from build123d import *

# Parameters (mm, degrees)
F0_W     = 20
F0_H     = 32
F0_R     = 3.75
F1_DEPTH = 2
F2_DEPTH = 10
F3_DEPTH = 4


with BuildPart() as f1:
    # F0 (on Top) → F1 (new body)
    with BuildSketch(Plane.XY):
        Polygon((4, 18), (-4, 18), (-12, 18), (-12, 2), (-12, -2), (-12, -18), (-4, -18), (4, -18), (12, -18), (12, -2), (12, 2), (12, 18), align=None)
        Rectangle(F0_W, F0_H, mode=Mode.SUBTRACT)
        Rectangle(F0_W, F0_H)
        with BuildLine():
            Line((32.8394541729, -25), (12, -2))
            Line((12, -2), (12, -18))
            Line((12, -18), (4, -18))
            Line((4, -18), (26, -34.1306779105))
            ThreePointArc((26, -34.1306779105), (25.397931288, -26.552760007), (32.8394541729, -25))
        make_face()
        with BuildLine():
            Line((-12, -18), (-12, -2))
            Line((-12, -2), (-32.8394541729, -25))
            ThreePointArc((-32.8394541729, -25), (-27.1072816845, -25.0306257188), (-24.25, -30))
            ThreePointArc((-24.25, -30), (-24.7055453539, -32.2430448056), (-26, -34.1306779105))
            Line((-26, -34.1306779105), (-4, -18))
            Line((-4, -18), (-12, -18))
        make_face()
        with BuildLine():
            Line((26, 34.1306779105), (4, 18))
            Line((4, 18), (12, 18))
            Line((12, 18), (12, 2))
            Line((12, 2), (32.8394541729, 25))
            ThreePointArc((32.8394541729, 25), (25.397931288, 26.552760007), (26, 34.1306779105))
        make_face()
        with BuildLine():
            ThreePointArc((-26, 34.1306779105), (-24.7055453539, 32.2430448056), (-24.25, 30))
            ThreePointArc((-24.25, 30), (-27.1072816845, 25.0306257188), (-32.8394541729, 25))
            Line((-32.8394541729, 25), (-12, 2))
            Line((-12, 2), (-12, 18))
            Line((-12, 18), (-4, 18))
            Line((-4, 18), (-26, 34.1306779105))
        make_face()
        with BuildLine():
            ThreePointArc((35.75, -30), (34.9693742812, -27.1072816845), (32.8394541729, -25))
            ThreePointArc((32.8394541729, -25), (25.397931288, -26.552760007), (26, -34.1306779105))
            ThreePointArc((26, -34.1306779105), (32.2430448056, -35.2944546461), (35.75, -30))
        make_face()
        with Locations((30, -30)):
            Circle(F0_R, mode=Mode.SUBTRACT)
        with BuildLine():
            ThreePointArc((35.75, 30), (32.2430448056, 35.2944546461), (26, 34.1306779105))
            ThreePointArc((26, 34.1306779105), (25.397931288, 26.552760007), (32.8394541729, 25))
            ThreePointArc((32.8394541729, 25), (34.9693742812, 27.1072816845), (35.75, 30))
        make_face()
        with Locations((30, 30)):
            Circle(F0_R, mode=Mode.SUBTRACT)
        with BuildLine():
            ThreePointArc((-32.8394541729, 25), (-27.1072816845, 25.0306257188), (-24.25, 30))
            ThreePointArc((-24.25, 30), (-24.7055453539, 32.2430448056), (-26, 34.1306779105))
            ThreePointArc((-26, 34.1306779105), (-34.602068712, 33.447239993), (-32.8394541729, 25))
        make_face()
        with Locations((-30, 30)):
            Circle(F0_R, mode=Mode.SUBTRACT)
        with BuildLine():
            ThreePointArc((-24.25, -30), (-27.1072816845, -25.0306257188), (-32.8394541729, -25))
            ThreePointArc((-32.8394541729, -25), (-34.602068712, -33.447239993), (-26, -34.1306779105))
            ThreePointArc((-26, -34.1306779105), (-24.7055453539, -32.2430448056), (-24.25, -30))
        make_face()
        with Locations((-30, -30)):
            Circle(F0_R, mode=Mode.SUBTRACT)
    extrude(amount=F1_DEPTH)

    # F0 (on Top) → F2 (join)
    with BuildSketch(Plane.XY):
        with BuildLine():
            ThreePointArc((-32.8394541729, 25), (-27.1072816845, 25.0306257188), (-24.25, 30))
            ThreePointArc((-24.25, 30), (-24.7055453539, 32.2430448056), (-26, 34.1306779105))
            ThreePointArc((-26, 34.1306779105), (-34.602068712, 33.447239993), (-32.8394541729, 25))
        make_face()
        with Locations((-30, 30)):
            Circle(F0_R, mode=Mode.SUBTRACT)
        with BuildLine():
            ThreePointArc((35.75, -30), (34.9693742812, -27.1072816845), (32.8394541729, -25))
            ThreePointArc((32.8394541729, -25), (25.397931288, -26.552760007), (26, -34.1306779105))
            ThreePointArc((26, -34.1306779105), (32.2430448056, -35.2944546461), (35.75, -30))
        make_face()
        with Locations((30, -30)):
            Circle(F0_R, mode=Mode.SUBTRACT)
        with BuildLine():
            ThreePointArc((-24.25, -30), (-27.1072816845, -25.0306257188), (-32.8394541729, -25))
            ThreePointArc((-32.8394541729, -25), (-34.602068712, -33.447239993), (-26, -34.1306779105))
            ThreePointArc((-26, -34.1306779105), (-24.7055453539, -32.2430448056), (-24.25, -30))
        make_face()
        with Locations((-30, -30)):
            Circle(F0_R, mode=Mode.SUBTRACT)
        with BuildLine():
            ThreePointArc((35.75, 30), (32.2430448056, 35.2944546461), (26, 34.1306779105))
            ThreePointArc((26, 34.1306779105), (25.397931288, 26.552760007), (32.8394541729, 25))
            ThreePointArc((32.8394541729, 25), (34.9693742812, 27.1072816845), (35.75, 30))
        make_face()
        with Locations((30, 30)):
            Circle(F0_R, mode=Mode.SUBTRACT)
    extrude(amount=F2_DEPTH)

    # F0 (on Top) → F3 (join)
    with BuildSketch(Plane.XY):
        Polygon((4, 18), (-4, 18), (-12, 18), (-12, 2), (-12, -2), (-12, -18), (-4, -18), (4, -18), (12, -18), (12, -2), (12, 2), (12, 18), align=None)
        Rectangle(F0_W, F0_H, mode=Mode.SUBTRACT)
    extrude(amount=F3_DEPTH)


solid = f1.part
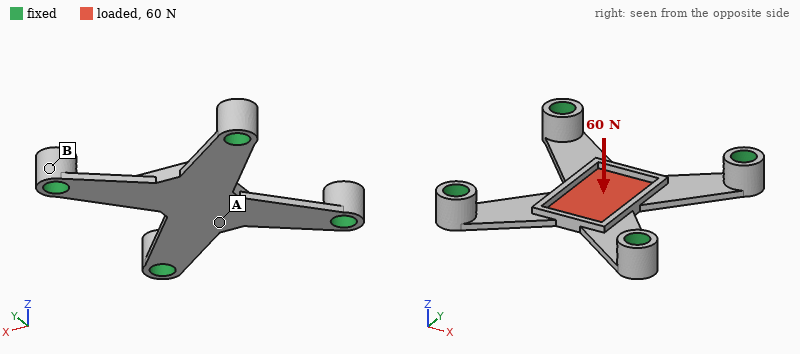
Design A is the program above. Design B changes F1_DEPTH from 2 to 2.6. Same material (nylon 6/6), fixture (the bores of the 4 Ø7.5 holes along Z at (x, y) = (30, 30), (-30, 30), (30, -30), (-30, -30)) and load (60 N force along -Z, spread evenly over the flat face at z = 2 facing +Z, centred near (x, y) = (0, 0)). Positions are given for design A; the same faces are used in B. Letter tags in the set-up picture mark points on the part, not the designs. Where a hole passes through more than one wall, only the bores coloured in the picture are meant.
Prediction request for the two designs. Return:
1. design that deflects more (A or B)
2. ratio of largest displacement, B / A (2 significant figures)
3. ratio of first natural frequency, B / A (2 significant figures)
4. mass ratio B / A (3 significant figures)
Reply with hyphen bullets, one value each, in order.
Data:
- A
- 0.59
- 1.2
- 1.16
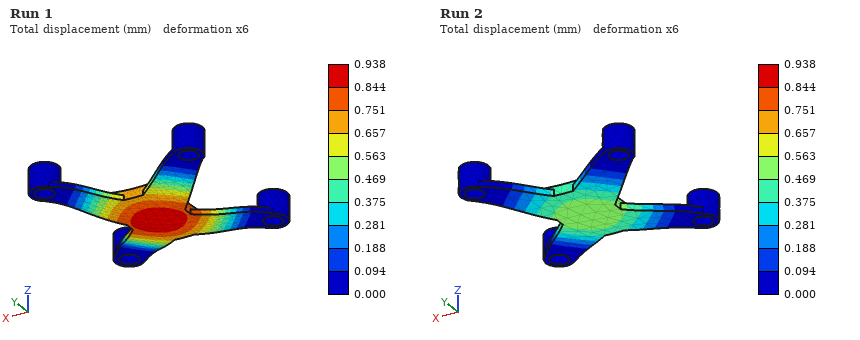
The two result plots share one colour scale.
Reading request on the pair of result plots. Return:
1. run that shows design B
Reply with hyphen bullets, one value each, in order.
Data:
- Run 2
